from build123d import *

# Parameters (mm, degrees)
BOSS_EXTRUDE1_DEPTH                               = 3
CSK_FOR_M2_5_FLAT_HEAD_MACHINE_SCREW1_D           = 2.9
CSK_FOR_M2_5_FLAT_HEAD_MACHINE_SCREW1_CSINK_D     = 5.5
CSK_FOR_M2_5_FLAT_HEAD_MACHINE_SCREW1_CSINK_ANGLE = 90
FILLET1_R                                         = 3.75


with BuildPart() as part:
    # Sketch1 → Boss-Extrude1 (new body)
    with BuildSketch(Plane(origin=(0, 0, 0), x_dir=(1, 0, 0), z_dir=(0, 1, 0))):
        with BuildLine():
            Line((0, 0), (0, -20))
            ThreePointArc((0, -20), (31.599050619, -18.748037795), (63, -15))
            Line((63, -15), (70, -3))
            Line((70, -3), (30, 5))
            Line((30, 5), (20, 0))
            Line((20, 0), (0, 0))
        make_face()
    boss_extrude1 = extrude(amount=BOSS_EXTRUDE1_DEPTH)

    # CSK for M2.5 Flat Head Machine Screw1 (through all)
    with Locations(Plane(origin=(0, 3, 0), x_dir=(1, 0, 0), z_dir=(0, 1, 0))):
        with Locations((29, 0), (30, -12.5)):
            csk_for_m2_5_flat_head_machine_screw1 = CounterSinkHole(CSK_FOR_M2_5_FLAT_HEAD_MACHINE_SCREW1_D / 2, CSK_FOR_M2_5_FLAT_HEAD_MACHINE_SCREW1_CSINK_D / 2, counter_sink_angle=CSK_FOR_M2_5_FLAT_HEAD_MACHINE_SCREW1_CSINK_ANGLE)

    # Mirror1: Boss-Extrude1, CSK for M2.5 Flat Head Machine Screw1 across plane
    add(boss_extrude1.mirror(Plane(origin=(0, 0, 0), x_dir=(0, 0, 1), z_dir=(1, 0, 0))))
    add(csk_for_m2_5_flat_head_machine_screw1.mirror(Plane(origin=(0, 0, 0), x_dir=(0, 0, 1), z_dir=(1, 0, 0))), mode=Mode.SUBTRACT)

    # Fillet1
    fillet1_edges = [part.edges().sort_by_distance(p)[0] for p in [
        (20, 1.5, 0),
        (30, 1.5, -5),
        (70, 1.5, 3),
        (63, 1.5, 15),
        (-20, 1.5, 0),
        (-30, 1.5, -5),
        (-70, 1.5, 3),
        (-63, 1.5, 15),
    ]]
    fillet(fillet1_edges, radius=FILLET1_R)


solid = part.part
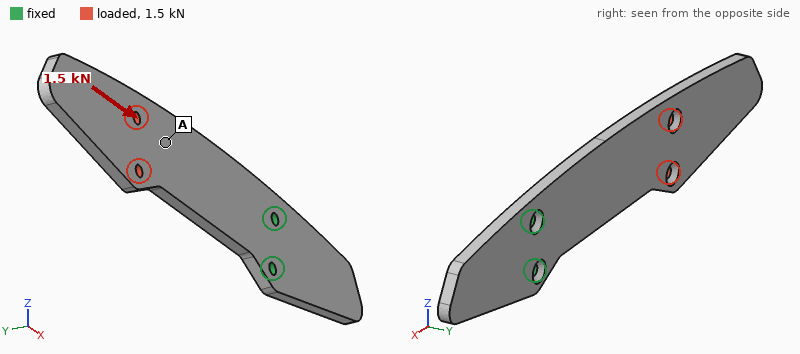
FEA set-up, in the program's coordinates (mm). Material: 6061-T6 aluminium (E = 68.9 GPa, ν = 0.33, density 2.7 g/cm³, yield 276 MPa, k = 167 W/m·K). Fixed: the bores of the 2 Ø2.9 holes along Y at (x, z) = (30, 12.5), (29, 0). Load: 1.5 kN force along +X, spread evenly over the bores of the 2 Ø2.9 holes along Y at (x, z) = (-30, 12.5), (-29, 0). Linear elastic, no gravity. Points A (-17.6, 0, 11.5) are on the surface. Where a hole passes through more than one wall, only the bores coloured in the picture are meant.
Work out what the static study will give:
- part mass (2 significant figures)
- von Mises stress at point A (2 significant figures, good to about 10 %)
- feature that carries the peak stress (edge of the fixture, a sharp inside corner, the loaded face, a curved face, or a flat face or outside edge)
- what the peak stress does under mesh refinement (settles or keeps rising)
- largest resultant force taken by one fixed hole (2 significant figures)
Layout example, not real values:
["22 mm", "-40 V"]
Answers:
["20 g", "51 MPa", "edge of the fixture", "keeps rising", "770 N"]
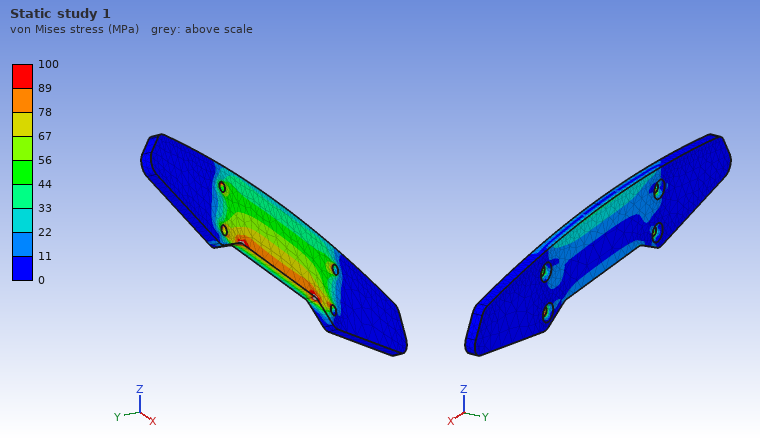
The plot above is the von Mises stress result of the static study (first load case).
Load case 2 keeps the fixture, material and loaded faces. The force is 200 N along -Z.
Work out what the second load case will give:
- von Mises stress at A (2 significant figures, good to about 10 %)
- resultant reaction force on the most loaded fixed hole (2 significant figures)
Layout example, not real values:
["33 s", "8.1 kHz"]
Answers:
["12 MPa", "880 N"]
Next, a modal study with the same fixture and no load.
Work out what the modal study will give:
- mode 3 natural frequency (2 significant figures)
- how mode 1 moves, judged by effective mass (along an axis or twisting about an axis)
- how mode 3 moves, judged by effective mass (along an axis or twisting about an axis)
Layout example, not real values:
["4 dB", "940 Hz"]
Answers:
["1800 Hz", "along Y", "along Z"]
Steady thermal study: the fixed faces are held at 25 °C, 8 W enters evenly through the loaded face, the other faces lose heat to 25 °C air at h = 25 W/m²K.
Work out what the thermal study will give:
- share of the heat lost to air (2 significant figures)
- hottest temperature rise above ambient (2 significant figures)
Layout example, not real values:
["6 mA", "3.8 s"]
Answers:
["32 %", "38 K"]
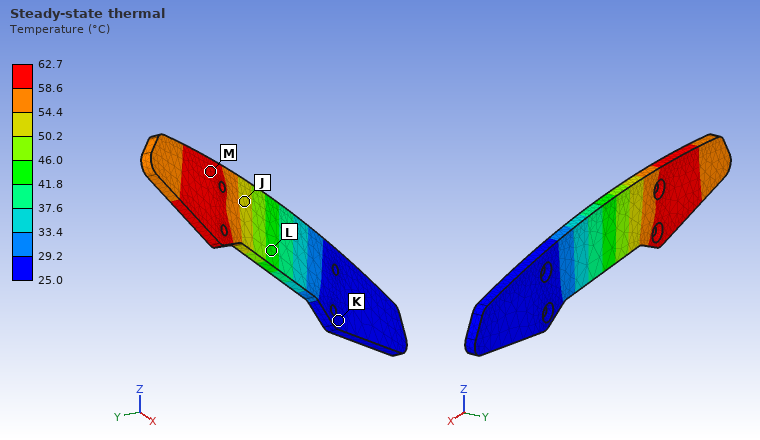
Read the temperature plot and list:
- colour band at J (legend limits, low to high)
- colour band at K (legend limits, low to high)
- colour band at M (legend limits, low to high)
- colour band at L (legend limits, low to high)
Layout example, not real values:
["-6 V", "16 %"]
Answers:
["50.2 to 54.4 °C", "25.0 to 29.2 °C", "58.6 to 62.7 °C", "41.8 to 46.0 °C"]
